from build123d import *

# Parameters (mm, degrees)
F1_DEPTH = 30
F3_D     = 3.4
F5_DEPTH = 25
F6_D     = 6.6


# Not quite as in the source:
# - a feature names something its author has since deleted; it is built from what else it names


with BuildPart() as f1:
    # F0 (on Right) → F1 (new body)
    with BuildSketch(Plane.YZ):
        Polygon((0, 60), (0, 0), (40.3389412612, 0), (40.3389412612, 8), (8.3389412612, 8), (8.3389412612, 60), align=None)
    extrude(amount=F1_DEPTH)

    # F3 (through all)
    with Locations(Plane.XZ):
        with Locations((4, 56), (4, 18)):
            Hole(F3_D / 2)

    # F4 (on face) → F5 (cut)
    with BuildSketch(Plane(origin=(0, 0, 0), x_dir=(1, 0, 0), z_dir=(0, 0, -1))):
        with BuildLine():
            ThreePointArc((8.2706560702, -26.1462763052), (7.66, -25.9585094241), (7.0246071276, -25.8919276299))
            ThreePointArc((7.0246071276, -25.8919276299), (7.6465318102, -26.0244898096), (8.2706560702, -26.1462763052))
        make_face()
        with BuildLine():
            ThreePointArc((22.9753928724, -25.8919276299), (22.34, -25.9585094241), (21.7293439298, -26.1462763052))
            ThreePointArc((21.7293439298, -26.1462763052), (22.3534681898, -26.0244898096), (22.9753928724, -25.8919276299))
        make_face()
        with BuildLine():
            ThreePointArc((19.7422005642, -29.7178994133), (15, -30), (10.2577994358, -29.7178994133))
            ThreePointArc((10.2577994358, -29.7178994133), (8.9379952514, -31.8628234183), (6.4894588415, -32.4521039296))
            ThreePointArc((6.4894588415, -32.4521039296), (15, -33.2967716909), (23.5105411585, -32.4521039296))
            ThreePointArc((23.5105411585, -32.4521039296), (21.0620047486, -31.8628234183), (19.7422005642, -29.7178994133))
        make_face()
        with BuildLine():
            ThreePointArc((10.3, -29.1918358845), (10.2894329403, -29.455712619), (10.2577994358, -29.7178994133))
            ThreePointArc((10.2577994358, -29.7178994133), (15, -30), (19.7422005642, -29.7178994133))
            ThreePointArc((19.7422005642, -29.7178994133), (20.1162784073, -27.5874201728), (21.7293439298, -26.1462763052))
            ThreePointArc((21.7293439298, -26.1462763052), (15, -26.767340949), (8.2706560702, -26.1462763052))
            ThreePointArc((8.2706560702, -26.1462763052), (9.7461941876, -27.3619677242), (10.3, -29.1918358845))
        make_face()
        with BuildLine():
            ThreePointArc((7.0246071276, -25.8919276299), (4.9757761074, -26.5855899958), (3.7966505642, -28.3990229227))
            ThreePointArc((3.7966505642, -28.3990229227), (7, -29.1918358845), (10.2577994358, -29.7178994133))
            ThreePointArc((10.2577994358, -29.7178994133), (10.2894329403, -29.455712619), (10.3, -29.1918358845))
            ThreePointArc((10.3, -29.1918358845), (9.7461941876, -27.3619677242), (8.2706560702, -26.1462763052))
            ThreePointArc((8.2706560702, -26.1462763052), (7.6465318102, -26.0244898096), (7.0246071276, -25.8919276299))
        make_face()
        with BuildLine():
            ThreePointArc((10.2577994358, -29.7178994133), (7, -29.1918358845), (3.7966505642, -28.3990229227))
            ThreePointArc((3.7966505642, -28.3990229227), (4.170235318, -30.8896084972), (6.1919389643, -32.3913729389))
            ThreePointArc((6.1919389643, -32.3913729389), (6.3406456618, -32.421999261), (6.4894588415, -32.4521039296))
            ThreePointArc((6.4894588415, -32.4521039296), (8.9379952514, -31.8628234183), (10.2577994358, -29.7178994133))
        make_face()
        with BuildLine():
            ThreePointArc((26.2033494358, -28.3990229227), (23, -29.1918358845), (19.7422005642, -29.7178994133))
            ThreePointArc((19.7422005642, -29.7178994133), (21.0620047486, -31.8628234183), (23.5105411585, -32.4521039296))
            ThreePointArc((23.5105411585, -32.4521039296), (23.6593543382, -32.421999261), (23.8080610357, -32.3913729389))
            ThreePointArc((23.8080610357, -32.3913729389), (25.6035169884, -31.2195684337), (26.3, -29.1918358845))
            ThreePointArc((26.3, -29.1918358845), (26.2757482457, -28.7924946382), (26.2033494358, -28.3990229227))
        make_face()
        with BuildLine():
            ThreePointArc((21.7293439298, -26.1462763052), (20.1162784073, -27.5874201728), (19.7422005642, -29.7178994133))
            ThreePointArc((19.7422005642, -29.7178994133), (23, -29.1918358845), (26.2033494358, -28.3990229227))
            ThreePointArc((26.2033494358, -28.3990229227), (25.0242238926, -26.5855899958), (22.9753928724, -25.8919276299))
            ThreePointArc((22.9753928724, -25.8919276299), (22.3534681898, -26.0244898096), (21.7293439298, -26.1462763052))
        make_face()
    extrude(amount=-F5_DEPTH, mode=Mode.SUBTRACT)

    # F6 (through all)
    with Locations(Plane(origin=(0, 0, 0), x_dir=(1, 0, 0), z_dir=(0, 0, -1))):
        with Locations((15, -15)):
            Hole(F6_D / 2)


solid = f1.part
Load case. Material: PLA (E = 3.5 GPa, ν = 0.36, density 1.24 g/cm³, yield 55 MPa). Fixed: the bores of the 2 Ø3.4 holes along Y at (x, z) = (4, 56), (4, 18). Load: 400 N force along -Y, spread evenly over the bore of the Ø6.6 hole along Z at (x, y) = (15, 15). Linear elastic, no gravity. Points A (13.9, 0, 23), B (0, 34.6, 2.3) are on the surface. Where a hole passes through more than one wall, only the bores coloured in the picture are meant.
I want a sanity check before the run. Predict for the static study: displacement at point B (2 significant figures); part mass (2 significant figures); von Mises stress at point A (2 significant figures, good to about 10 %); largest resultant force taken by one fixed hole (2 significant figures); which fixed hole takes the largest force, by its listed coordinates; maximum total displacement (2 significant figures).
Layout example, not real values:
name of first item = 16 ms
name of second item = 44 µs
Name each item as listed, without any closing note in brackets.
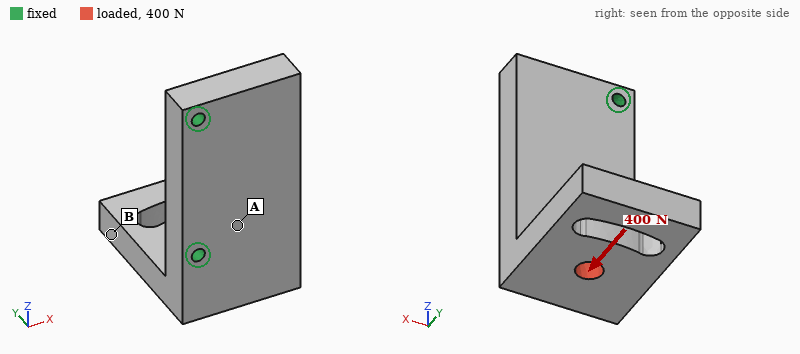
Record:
displacement at point B = 0.53 mm
part mass = 26 g
von Mises stress at point A = 8.8 MPa
largest resultant force taken by one fixed hole = 460 N
which fixed hole takes the largest force, by its listed coordinates = (4, 18)
maximum total displacement = 0.79 mm
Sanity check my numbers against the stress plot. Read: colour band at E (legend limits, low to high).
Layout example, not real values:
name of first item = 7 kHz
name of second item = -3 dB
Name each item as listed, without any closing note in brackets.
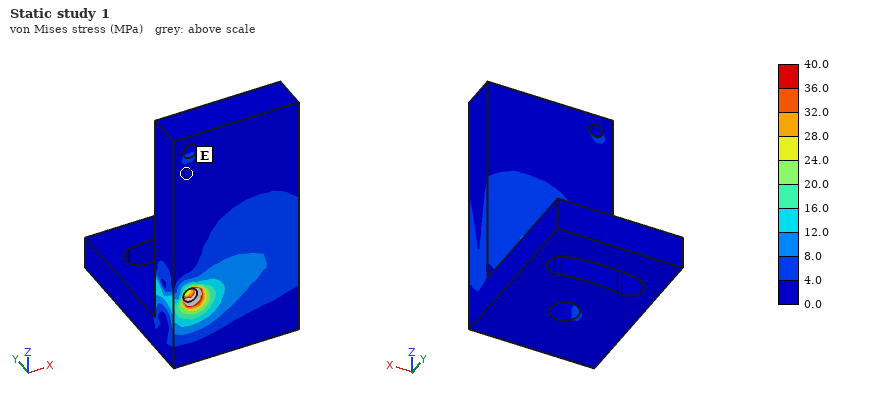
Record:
colour band at E = 0.0 to 4.0 MPa
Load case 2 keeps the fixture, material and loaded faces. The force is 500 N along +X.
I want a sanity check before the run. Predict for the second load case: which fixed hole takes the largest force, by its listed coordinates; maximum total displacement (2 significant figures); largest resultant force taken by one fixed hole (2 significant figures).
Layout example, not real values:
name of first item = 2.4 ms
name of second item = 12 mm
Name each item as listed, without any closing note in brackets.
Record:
which fixed hole takes the largest force, by its listed coordinates = (4, 18)
maximum total displacement = 0.82 mm
largest resultant force taken by one fixed hole = 680 N
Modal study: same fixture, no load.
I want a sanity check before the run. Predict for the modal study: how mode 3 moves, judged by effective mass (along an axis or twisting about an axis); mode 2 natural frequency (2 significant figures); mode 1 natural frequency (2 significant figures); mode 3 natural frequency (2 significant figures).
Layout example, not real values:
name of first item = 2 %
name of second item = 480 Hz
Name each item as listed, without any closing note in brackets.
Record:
how mode 3 moves, judged by effective mass = along Y
mode 2 natural frequency = 1200 Hz
mode 1 natural frequency = 990 Hz
mode 3 natural frequency = 2800 Hz
